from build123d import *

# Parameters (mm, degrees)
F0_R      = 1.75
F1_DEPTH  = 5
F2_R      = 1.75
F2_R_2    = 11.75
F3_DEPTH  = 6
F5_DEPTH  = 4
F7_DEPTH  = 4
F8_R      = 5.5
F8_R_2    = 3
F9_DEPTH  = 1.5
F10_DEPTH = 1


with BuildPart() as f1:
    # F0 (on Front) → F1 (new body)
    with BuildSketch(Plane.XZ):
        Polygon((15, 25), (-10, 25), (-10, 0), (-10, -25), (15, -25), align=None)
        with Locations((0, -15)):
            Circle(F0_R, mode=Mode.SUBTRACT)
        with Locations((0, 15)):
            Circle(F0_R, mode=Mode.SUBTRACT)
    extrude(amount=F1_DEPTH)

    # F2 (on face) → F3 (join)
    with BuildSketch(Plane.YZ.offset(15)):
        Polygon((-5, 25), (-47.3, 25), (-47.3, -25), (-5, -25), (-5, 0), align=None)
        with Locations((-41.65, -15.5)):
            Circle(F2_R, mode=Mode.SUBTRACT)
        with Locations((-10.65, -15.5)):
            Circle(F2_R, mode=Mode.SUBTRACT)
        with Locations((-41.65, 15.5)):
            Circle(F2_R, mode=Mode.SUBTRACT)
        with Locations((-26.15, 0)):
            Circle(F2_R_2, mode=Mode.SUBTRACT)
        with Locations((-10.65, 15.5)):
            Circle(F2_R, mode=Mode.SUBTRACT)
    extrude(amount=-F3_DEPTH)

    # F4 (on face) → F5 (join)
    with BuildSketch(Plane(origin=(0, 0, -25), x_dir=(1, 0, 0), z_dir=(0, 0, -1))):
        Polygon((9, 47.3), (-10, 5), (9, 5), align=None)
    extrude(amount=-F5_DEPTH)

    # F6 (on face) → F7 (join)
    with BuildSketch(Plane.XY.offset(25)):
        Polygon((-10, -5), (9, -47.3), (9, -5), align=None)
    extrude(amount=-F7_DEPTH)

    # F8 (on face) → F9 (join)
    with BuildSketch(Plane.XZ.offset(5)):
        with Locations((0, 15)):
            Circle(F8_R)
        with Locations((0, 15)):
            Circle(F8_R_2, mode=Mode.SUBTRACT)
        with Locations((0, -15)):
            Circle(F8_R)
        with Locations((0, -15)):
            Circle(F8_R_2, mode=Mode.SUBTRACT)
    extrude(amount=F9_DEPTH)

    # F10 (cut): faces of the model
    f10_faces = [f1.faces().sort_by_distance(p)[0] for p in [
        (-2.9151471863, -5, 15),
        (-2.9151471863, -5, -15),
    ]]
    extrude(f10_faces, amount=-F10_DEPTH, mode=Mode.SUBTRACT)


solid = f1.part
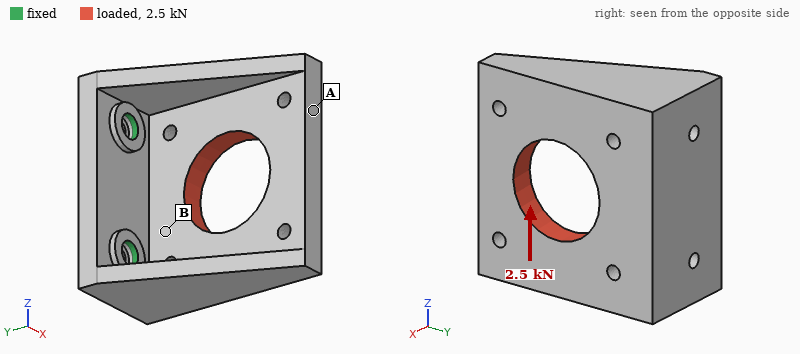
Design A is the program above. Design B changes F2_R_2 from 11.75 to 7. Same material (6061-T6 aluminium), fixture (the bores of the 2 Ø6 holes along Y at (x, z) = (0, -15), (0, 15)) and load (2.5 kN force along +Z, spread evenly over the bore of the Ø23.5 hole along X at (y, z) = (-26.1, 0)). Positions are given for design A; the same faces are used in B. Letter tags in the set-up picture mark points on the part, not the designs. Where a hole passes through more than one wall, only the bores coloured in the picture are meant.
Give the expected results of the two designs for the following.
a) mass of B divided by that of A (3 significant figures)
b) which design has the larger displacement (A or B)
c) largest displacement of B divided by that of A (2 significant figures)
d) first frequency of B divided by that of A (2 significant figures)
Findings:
1.09
A
0.87
0.95
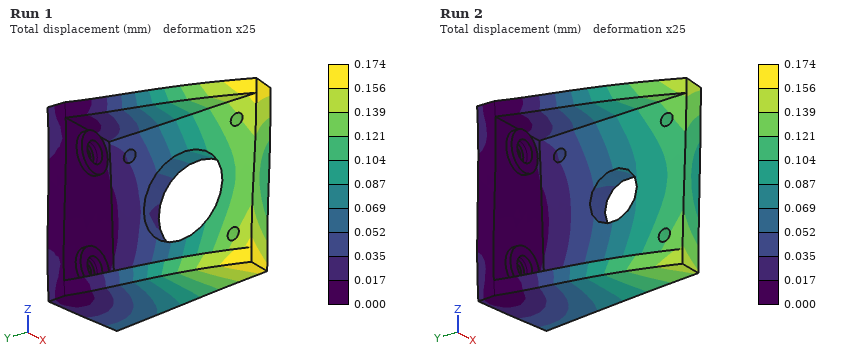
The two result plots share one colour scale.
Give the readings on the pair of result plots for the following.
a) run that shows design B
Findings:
Run 2
